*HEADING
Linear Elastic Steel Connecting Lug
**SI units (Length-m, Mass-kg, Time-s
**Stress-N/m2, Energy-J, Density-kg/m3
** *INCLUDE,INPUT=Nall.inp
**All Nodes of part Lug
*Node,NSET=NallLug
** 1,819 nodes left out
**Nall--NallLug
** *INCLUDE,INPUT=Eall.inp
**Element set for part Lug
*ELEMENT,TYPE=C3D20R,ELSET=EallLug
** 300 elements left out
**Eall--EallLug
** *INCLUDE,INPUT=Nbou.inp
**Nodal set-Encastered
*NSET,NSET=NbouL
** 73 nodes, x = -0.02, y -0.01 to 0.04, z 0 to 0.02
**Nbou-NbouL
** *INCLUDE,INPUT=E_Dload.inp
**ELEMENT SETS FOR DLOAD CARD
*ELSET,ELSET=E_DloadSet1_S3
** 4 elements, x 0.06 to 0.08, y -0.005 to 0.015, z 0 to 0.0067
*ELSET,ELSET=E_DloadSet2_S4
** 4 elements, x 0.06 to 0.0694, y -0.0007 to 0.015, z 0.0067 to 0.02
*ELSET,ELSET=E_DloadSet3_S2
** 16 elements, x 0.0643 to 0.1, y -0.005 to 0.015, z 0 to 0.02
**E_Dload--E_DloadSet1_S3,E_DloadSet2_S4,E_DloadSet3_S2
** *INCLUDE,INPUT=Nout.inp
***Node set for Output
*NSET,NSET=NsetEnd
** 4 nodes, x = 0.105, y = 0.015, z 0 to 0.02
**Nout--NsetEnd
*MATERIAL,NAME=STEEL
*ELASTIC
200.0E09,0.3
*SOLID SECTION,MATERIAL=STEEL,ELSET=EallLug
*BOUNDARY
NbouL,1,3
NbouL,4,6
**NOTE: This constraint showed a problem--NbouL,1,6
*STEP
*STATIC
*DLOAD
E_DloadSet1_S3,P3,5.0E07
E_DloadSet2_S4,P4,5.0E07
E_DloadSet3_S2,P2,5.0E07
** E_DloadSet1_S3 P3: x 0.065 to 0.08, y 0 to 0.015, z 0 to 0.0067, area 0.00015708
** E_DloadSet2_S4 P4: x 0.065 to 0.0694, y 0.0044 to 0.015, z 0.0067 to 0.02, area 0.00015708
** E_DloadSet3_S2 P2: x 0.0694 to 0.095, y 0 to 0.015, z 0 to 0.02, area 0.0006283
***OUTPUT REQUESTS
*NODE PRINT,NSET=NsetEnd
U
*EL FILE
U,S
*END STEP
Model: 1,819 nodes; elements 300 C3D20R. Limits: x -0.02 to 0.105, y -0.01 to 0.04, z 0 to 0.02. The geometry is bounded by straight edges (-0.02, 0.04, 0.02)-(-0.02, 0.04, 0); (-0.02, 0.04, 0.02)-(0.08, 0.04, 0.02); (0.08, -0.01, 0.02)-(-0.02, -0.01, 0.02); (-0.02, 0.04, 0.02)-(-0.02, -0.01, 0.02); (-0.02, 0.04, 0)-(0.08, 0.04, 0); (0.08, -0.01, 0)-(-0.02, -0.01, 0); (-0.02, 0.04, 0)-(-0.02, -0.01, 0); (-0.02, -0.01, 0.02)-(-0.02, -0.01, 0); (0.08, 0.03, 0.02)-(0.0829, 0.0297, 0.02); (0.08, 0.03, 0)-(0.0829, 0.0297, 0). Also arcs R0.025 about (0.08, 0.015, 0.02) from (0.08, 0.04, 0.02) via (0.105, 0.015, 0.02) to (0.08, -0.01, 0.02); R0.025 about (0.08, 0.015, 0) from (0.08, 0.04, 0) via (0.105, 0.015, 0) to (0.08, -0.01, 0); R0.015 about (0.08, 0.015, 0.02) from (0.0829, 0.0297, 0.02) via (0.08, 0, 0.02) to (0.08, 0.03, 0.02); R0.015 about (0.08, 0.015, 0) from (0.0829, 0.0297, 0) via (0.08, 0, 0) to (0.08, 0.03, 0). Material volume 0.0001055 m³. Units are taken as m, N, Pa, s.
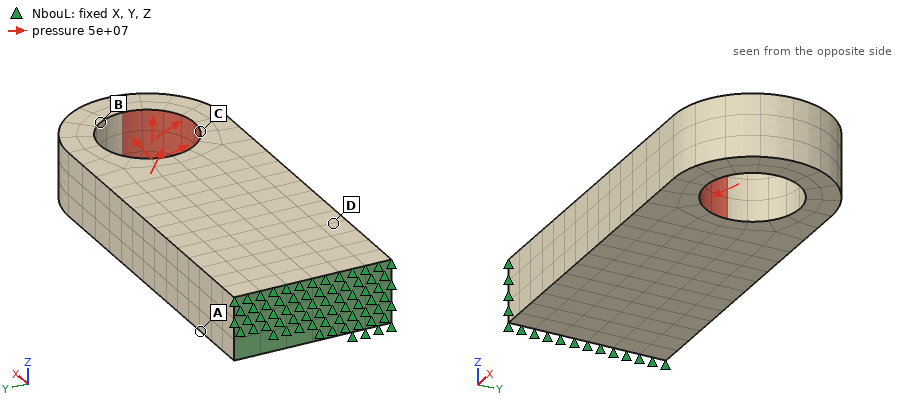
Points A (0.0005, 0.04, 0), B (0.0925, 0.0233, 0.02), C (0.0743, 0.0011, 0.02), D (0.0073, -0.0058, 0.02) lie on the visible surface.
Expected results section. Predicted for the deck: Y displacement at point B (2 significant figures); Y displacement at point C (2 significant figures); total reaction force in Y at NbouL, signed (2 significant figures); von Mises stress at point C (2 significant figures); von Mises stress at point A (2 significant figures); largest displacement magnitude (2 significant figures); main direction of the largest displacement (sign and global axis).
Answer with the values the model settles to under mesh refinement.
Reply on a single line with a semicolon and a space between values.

-3.8e-04 m; -2.8e-04 m; 30000 N; 2.7e+08 Pa; 2.8e+08 Pa; 4.2e-04 m; -Y
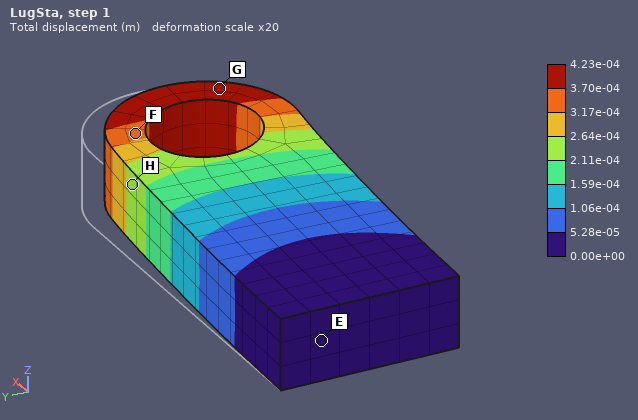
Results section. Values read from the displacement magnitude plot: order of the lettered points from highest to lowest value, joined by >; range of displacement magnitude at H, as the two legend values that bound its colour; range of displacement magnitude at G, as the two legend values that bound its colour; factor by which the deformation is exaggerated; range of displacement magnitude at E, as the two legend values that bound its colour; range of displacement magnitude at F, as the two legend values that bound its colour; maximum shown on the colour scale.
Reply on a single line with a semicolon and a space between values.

G > F > H > E; 2.11e-04 to 2.64e-04 m; 3.70e-04 to 4.23e-04 m; 20; 0.00e+00 to 5.28e-05 m; 3.17e-04 to 3.70e-04 m; 4.23e-04 m
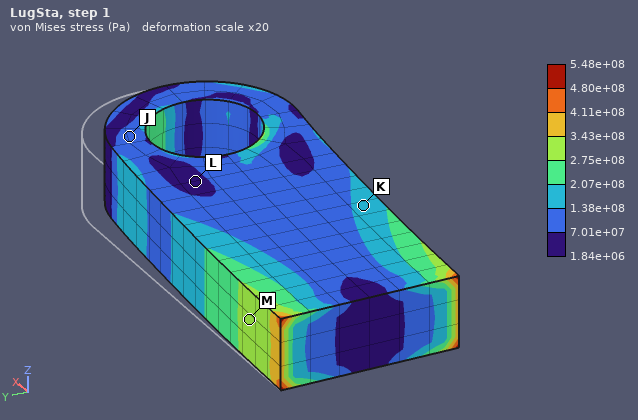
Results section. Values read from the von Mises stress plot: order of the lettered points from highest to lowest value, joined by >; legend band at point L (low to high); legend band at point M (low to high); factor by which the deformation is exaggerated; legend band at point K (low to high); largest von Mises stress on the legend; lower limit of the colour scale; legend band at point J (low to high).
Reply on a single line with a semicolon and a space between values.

M > K > J > L; 1.84e+06 to 7.01e+07 Pa; 2.75e+08 to 3.43e+08 Pa; 20; 1.38e+08 to 2.07e+08 Pa; 5.48e+08 Pa; 1.84e+06 Pa; 7.01e+07 to 1.38e+08 Pa
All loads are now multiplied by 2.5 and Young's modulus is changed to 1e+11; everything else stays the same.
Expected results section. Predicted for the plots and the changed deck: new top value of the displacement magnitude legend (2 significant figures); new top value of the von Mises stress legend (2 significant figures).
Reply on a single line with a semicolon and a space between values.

0.0021 m; 1.4e+09 Pa
